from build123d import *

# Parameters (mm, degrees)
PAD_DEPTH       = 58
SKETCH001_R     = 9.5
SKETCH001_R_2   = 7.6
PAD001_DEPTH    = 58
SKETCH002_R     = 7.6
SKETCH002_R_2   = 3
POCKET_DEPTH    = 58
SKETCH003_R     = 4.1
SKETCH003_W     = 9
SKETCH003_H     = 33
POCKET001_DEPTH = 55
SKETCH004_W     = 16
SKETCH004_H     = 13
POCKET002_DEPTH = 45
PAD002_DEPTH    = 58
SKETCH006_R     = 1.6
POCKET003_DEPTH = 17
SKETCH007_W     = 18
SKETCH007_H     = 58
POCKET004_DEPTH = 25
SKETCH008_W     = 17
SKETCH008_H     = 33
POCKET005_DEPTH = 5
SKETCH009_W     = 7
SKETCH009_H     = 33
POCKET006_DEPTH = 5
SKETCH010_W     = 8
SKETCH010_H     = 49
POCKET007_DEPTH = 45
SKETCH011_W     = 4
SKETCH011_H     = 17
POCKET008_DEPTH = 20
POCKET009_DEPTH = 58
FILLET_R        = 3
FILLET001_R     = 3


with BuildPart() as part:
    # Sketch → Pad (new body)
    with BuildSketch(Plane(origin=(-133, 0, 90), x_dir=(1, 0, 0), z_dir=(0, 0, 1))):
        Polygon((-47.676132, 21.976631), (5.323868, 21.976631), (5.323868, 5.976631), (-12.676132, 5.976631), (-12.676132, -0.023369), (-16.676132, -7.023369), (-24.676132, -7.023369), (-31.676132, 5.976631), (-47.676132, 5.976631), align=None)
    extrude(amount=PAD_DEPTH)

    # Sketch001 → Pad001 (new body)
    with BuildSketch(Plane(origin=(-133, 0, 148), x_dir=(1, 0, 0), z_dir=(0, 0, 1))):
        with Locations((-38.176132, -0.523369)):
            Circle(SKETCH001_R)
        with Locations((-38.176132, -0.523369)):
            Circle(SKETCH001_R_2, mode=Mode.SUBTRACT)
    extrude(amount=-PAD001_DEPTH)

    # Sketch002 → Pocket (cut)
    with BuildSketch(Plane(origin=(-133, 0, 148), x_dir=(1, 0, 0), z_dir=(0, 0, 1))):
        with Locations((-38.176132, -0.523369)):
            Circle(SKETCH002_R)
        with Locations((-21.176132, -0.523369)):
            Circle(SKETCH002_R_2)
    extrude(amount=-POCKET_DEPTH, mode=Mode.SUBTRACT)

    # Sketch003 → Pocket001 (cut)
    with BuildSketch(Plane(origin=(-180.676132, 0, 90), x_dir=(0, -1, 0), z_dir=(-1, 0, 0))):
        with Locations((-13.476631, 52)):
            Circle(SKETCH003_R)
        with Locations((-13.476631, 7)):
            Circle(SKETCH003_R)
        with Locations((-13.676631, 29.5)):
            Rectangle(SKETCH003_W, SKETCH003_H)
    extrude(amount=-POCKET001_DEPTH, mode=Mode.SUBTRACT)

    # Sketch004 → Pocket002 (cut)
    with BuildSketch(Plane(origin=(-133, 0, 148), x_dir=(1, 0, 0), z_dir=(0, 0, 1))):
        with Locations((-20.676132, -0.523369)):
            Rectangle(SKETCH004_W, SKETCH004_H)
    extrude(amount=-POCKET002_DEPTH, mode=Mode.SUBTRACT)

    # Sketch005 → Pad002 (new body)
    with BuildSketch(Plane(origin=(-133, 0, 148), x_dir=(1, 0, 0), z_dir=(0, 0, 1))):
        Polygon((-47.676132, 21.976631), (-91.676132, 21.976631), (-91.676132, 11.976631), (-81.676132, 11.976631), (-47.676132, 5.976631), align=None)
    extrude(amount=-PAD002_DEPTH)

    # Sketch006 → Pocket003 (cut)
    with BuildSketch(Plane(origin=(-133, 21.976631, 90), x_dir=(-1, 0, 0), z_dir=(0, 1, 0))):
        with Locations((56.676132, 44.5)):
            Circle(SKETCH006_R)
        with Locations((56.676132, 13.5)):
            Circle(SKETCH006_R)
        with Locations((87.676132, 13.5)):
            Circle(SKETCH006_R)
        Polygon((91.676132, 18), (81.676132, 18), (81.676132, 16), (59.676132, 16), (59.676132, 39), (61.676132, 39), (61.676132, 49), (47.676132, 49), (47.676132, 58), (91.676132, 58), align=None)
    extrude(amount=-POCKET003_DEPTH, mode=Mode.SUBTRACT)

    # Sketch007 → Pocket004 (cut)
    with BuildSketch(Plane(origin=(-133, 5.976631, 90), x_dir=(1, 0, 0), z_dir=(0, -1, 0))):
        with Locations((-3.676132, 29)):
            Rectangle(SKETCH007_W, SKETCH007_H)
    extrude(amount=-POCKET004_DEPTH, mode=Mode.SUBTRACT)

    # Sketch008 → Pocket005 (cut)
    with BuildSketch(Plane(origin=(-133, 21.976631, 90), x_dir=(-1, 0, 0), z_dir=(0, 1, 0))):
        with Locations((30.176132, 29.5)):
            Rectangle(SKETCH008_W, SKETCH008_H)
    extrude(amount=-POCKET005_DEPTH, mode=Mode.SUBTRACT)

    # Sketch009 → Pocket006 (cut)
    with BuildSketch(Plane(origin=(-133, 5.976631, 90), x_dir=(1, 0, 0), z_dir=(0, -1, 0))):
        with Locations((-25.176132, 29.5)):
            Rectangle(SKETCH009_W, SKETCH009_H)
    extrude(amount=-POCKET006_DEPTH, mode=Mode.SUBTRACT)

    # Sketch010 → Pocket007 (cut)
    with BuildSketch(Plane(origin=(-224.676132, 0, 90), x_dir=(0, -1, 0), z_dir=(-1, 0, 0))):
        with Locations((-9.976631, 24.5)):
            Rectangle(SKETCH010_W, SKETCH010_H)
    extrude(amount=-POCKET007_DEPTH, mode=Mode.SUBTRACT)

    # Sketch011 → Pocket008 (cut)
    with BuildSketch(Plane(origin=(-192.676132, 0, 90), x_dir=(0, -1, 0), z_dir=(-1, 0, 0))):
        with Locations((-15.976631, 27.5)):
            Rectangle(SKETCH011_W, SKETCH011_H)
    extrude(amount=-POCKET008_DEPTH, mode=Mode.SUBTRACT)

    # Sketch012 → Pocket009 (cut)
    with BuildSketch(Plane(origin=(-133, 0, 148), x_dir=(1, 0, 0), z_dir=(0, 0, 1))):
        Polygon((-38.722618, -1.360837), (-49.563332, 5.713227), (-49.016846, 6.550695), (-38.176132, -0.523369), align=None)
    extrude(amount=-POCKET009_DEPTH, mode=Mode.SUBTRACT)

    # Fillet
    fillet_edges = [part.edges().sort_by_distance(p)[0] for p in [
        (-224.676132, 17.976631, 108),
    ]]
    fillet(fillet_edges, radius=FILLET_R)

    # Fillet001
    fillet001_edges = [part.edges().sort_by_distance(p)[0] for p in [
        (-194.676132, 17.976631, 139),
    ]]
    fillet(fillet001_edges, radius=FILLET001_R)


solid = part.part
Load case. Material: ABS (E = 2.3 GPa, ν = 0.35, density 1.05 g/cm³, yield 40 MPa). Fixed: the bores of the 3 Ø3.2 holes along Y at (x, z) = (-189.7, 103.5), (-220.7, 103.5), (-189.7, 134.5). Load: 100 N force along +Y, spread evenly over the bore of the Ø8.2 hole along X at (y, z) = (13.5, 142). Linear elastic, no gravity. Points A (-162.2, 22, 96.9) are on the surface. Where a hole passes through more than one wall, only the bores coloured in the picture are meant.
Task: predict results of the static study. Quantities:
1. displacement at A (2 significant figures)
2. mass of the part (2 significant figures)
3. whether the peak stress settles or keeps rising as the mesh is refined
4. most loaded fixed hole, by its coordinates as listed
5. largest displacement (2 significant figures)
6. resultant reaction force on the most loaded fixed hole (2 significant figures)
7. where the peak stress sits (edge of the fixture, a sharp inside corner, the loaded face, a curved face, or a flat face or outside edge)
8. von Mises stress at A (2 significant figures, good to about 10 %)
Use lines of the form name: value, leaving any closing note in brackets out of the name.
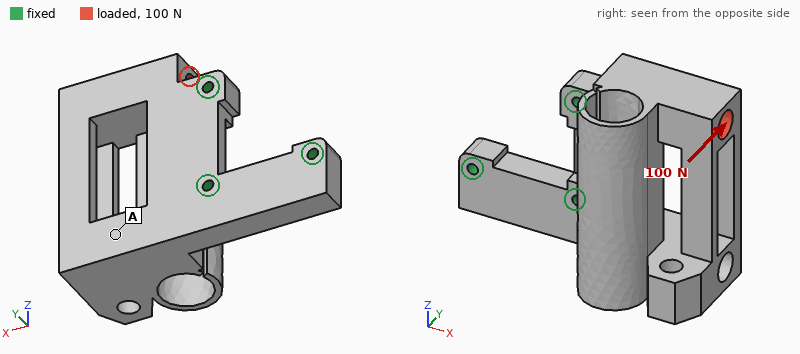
displacement at A: 0.19 mm
mass of the part: 31 g
whether the peak stress settles or keeps rising as the mesh is refined: keeps rising
most loaded fixed hole, by its coordinates as listed: (-189.7, 134.5)
largest displacement: 1.1 mm
resultant reaction force on the most loaded fixed hole: 100 N
where the peak stress sits: a sharp inside corner
von Mises stress at A: 1.5 MPa
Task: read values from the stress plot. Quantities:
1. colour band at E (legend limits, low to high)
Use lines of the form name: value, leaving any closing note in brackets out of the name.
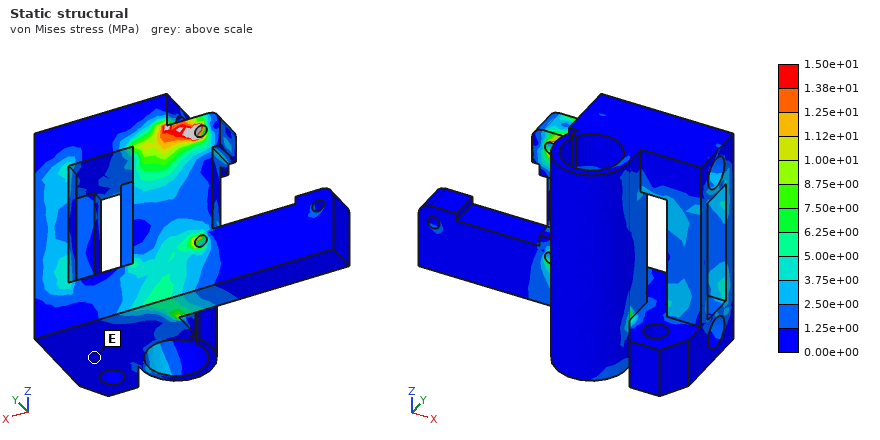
colour band at E: 0.00e+00 to 1.25e+00 MPa
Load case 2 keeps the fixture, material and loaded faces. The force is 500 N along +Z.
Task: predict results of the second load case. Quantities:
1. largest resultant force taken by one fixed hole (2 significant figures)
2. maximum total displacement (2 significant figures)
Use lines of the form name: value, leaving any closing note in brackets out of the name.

largest resultant force taken by one fixed hole: 400 N
maximum total displacement: 0.53 mm
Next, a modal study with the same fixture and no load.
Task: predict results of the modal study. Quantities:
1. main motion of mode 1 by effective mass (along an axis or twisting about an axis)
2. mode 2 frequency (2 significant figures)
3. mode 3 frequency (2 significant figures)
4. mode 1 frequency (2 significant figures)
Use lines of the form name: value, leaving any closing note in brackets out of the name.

main motion of mode 1 by effective mass: along Y
mode 2 frequency: 570 Hz
mode 3 frequency: 720 Hz
mode 1 frequency: 460 Hz
